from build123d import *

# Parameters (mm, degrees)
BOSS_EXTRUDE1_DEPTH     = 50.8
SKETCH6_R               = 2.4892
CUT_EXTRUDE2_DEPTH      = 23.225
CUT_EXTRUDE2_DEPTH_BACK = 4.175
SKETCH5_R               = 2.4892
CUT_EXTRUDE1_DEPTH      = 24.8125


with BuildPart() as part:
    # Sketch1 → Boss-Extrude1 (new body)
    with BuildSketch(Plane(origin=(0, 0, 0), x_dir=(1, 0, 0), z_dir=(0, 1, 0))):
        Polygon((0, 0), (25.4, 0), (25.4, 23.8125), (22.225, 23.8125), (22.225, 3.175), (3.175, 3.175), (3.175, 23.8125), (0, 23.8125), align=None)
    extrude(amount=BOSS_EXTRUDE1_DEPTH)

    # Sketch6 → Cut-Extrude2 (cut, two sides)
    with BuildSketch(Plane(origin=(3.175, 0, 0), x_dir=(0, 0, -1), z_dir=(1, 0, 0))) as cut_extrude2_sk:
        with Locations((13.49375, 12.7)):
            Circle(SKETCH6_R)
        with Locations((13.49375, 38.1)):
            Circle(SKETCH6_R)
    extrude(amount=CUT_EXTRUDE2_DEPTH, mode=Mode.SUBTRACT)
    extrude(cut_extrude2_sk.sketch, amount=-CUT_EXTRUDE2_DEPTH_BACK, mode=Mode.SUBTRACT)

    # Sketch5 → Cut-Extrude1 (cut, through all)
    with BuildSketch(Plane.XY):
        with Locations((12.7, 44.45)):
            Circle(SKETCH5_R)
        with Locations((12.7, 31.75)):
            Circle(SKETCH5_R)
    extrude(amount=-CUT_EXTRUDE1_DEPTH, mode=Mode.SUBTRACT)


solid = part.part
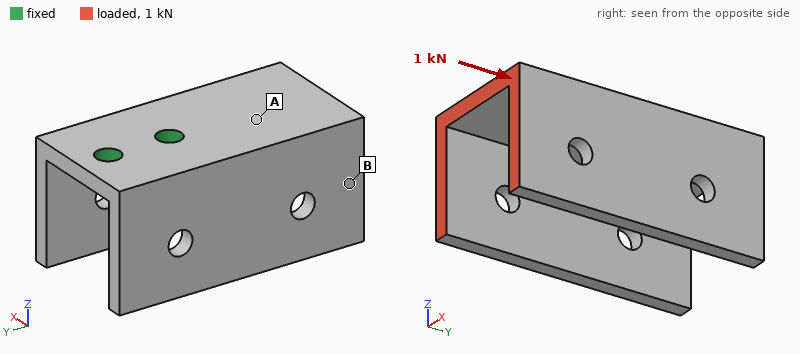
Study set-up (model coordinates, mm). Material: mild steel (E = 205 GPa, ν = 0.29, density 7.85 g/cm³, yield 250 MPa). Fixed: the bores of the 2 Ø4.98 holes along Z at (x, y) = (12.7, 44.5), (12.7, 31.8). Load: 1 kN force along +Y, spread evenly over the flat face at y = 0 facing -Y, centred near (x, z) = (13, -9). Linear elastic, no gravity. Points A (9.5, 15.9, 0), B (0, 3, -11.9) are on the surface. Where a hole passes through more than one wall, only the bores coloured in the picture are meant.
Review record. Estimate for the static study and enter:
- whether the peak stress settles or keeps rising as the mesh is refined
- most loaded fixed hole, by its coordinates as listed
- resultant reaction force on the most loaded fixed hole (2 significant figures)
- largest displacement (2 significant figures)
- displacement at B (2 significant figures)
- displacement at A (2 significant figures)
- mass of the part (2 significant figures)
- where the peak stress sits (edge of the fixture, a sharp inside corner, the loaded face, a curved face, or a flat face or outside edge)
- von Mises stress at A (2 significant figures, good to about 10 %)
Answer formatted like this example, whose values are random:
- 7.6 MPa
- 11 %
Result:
- keeps rising
- (12.7, 31.8)
- 780 N
- 21 µm
- 17 µm
- 8.0 µm
- 82 g
- edge of the fixture
- 14 MPa
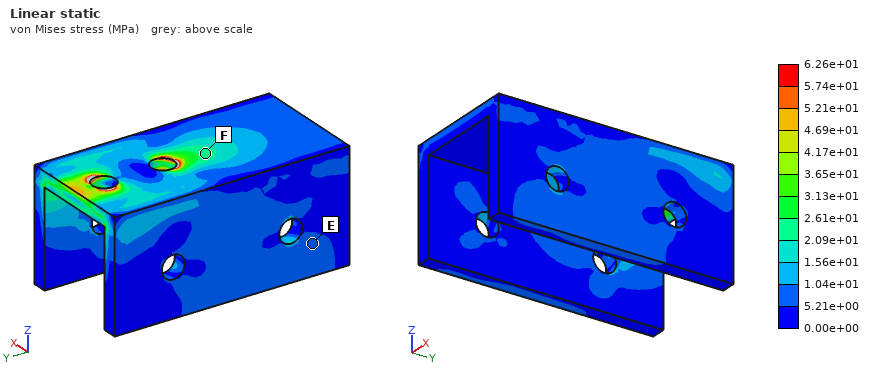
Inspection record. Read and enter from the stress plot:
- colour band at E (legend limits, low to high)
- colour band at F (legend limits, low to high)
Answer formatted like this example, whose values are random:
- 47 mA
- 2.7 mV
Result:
- 5.21e+00 to 1.04e+01 MPa
- 2.09e+01 to 2.61e+01 MPa
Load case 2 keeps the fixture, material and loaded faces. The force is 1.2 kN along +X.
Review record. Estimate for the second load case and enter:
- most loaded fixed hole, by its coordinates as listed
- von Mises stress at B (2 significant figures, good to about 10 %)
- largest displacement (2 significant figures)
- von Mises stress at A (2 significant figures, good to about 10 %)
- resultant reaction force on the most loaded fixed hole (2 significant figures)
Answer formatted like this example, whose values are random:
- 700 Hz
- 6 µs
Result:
- (12.7, 31.8)
- 82 MPa
- 0.19 mm
- 27 MPa
- 3.1 kN
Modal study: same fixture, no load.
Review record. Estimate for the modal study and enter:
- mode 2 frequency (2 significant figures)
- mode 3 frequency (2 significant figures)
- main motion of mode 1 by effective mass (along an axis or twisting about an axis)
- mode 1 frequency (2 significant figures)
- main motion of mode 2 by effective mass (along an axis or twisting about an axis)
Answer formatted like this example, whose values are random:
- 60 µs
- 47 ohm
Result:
- 3000 Hz
- 3500 Hz
- along X
- 2300 Hz
- along Z
